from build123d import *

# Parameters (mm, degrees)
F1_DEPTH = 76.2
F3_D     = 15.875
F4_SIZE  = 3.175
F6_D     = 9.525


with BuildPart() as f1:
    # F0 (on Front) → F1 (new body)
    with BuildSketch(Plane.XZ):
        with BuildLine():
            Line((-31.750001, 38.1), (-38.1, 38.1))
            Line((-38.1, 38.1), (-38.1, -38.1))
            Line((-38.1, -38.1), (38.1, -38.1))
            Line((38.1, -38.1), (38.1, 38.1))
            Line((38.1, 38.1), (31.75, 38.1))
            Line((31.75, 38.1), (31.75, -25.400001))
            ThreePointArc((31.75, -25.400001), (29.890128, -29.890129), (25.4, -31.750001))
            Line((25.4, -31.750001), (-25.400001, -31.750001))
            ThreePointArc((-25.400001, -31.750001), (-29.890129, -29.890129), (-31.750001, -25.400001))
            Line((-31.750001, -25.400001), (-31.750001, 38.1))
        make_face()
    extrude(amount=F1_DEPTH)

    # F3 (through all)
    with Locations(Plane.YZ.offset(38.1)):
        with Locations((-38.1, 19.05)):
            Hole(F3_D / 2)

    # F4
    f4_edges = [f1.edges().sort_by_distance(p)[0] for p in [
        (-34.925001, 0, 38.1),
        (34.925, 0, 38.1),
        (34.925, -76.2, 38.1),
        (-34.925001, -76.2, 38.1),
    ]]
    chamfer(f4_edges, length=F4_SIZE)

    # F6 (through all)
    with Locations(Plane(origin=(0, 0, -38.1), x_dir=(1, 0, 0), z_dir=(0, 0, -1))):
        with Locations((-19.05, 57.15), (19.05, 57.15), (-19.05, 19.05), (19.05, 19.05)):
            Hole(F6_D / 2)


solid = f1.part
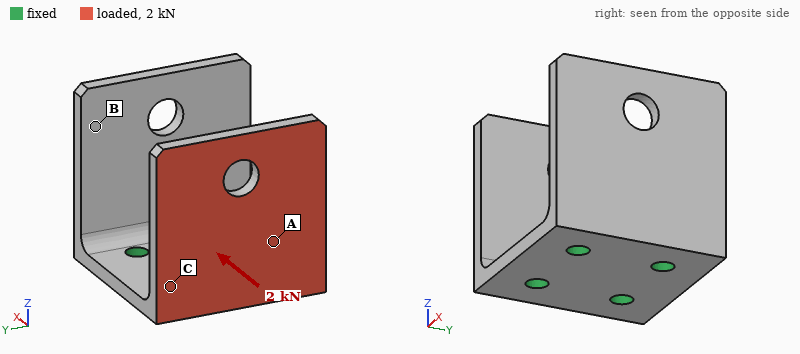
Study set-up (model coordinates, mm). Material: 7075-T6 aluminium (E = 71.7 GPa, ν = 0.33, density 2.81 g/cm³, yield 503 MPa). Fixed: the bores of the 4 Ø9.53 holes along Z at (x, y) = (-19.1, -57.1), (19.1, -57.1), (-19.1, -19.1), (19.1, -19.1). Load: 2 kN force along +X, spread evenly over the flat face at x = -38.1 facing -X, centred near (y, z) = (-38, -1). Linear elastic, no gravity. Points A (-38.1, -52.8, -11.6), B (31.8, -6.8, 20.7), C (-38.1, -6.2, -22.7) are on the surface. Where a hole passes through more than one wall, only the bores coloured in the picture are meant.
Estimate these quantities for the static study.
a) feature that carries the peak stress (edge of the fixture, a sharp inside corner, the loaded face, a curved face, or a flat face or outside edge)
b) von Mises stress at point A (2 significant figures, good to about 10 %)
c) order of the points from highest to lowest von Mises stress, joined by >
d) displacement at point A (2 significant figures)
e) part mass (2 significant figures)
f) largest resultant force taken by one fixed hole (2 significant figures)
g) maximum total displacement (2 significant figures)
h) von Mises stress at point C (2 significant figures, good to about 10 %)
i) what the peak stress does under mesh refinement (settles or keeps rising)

edge of the fixture
55 MPa
C > A > B
0.23 mm
280 g
930 N
1.0 mm
83 MPa
keeps rising
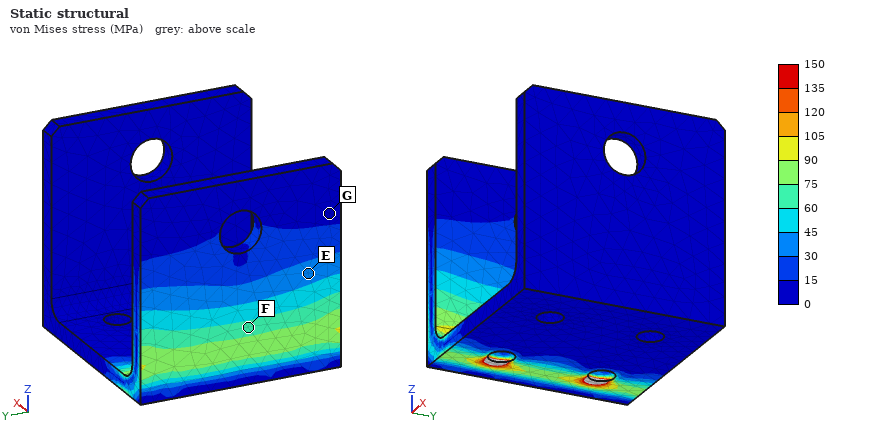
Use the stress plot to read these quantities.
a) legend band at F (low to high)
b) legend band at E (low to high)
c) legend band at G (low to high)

60 to 75 MPa
30 to 45 MPa
0 to 15 MPa
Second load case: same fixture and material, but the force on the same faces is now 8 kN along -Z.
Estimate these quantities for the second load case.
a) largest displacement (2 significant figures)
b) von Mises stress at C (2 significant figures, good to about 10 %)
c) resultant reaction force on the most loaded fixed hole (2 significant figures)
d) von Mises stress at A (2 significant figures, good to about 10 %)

0.93 mm
47 MPa
4.3 kN
41 MPa
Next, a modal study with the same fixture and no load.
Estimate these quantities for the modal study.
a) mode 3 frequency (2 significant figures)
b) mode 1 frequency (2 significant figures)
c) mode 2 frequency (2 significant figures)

2000 Hz
880 Hz
890 Hz
